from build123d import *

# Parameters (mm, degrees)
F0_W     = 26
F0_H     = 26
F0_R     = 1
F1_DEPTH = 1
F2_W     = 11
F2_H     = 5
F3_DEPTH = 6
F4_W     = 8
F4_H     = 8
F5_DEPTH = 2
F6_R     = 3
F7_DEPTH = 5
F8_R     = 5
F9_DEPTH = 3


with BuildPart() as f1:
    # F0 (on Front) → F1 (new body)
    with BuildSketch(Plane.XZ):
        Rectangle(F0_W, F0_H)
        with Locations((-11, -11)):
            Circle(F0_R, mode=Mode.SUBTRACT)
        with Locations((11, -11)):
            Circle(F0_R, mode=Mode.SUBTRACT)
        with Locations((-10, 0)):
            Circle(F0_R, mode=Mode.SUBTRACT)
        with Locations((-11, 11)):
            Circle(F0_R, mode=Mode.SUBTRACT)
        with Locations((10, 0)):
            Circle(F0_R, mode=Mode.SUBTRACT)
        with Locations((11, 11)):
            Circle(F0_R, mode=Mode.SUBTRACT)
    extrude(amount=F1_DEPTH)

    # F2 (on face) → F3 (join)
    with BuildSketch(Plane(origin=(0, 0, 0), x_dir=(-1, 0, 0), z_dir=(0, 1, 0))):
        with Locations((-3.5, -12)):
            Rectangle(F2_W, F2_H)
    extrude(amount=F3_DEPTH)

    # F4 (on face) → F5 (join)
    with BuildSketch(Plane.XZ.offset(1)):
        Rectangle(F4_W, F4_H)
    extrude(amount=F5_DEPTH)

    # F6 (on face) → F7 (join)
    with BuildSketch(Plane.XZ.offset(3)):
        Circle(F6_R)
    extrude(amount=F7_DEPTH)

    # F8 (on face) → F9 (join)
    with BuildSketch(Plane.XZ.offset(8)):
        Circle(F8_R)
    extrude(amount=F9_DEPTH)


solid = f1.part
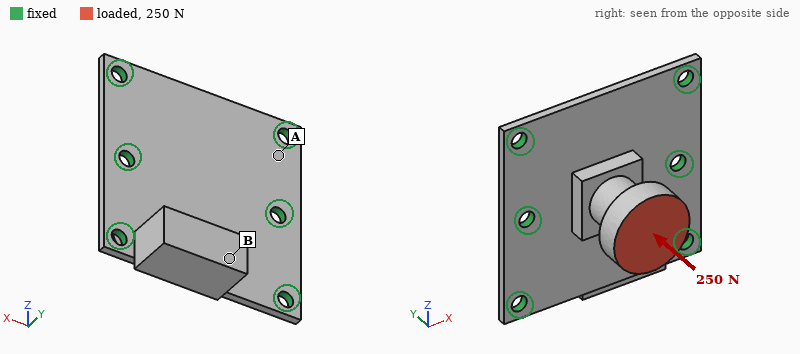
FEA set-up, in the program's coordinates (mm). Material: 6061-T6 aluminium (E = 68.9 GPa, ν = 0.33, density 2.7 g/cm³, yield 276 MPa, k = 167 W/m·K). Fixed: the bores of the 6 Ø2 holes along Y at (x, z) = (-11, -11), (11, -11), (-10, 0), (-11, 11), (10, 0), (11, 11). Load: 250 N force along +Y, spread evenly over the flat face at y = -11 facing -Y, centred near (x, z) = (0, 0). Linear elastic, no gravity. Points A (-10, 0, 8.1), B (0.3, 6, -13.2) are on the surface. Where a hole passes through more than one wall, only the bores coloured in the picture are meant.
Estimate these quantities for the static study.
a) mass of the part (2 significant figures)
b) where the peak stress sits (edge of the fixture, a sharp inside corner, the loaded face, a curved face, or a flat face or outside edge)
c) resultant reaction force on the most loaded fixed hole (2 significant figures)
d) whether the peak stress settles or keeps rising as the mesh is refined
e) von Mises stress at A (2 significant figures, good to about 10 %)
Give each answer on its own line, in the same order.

4.0 g
edge of the fixture
110 N
keeps rising
38 MPa
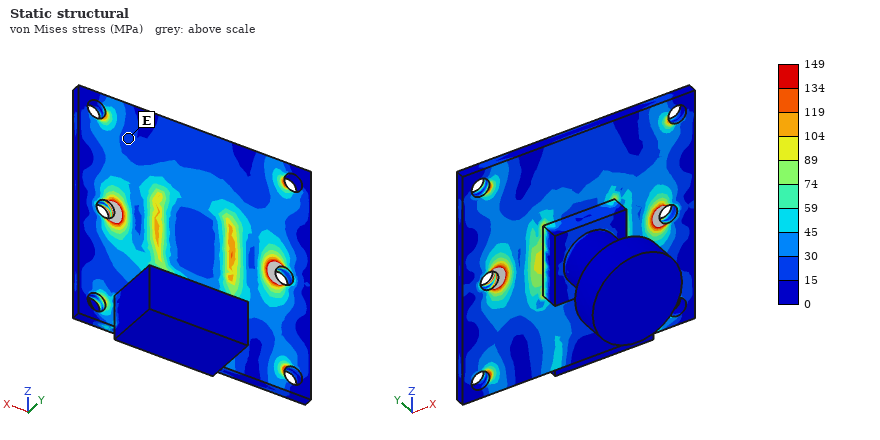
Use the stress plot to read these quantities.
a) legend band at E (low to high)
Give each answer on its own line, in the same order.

15 to 30 MPa
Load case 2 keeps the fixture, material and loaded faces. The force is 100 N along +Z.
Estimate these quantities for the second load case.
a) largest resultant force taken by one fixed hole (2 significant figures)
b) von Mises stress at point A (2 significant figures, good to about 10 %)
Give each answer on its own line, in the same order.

31 N
35 MPa
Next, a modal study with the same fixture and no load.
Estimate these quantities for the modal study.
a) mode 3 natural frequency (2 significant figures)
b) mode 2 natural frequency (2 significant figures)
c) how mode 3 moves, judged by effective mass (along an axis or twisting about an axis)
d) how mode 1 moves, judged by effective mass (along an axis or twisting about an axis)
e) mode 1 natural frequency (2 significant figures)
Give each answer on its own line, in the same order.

9000 Hz
7900 Hz
along Y
along Z
6400 Hz
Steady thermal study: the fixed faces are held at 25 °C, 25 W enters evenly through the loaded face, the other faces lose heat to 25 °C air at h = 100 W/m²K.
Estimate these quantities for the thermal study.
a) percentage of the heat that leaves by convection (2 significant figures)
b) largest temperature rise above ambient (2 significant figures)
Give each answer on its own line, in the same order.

13 %
71 K
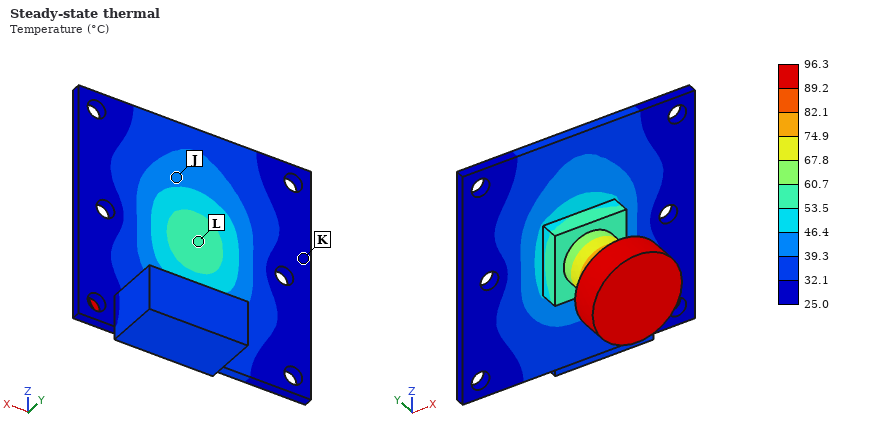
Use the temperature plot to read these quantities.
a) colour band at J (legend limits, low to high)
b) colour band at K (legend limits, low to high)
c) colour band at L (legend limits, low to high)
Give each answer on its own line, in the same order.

39.3 to 46.4 °C
25.0 to 32.1 °C
53.5 to 60.7 °C
